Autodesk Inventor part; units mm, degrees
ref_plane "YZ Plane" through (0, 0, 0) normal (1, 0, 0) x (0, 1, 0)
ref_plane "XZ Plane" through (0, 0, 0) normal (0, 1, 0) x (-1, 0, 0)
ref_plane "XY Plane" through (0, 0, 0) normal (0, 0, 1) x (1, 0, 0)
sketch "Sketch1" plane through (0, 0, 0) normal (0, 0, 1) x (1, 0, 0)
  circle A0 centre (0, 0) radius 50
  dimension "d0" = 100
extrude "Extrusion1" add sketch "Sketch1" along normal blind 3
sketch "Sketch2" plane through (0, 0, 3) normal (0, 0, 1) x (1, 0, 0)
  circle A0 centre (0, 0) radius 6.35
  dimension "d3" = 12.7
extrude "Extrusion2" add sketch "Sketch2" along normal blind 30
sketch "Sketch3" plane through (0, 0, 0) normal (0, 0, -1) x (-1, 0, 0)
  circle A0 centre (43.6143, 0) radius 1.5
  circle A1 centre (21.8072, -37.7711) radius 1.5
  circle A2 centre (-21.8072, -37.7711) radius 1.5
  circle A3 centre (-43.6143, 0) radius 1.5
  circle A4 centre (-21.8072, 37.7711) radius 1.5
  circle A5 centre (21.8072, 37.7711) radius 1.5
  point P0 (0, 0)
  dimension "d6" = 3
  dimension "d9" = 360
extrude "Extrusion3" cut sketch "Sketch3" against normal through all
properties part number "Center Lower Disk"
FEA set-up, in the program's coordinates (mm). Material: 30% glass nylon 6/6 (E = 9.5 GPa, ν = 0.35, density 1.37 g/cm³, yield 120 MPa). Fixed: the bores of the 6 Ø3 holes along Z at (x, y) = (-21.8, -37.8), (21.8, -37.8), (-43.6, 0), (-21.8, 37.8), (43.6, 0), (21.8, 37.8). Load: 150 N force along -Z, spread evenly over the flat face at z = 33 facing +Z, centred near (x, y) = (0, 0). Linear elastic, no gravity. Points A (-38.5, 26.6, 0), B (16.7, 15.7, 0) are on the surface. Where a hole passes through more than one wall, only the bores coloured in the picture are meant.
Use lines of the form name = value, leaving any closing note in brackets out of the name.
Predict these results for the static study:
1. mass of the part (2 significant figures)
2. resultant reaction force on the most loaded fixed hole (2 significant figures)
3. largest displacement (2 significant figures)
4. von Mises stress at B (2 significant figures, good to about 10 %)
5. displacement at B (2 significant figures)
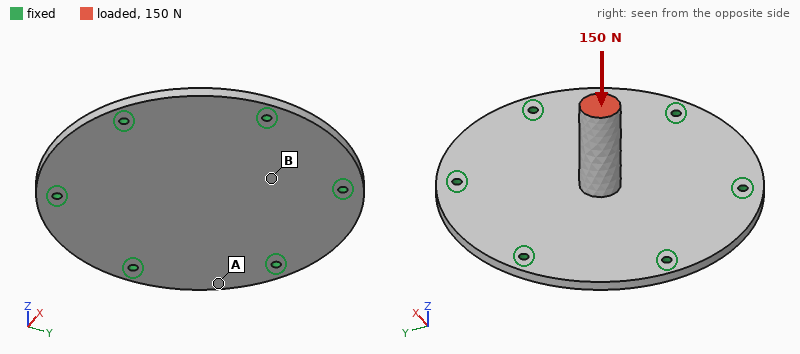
mass of the part = 37 g
resultant reaction force on the most loaded fixed hole = 25 N
largest displacement = 0.23 mm
von Mises stress at B = 5.0 MPa
displacement at B = 0.12 mm
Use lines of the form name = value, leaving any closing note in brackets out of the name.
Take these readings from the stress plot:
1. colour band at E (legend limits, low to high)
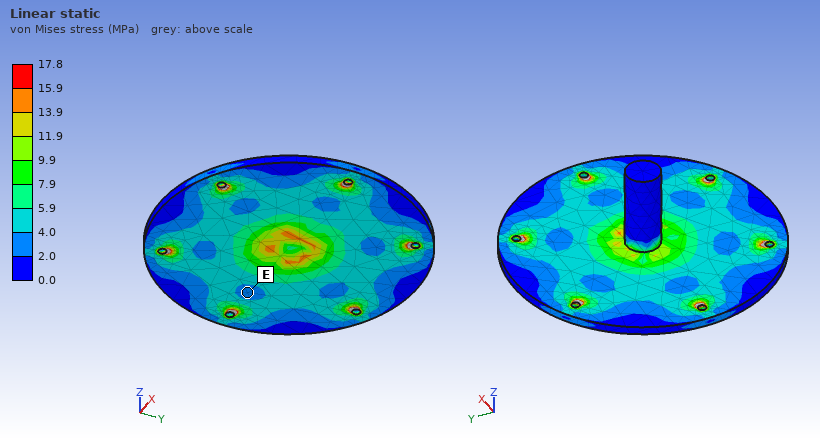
colour band at E = 2.0 to 4.0 MPa
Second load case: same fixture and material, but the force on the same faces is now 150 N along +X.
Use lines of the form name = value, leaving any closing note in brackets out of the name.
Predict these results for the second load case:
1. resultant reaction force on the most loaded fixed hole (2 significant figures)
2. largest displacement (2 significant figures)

resultant reaction force on the most loaded fixed hole = 60 N
largest displacement = 0.78 mm
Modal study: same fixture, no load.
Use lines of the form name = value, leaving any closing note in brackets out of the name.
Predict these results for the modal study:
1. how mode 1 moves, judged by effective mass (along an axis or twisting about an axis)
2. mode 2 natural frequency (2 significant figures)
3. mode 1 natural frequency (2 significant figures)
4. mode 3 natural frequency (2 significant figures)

how mode 1 moves, judged by effective mass = along Z
mode 2 natural frequency = 1600 Hz
mode 1 natural frequency = 1200 Hz
mode 3 natural frequency = 1600 Hz
